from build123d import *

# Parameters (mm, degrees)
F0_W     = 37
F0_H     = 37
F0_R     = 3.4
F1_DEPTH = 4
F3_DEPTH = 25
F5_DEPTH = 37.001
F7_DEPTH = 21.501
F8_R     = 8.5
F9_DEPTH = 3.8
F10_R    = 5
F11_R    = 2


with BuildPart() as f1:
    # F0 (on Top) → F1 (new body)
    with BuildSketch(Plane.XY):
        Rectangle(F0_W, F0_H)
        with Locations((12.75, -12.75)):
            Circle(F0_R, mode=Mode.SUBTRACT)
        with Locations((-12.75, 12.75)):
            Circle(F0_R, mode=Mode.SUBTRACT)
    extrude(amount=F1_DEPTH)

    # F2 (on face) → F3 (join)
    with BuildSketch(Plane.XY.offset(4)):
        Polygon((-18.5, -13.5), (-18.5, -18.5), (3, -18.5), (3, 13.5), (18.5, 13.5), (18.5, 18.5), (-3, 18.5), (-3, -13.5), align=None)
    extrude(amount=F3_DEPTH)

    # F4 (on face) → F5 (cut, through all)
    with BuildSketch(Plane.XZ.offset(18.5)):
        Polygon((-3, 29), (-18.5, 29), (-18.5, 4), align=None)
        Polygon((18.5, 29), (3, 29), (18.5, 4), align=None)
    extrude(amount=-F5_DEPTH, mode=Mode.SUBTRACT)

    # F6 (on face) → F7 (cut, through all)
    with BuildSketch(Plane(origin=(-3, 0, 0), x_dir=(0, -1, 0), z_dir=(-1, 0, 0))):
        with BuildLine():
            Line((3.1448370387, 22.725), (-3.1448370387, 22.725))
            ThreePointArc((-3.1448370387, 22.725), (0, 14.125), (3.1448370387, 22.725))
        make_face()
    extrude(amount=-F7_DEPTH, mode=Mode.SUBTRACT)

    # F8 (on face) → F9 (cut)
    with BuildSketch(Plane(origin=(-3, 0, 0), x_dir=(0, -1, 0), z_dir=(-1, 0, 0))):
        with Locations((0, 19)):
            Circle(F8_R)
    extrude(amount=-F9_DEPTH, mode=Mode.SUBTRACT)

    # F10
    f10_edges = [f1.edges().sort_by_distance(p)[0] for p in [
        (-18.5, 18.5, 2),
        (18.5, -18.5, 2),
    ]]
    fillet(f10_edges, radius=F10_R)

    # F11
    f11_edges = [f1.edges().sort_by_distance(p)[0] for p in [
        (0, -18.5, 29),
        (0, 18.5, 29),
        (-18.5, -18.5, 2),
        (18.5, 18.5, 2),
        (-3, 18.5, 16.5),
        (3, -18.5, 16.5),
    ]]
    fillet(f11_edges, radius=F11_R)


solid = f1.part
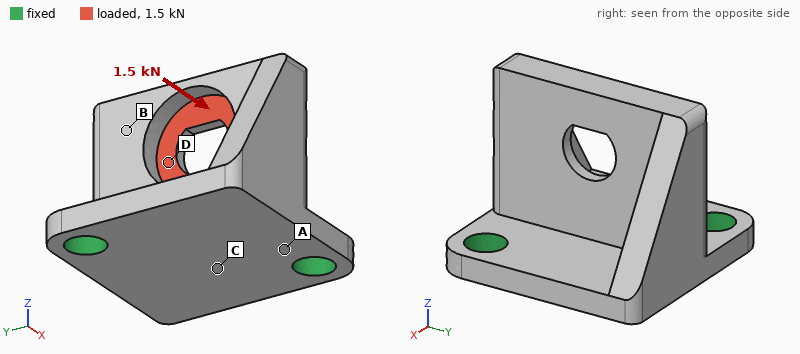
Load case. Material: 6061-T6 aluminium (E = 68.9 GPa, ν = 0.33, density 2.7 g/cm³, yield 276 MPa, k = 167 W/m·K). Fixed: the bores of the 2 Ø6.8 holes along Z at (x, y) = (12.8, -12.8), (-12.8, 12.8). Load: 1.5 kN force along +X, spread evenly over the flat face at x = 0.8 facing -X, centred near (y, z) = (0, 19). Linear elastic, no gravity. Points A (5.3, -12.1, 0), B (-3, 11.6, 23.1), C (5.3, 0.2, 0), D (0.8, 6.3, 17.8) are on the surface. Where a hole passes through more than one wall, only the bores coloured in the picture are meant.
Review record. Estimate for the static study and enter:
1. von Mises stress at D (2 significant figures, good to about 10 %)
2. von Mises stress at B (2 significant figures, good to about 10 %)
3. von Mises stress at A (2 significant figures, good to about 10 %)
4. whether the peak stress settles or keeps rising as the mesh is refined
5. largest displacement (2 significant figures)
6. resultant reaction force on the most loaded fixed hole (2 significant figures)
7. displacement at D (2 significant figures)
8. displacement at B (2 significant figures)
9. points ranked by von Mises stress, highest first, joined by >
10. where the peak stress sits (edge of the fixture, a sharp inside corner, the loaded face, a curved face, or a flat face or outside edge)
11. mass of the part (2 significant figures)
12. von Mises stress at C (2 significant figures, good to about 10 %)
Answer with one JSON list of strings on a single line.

["41 MPa", "21 MPa", "110 MPa", "keeps rising", "0.27 mm", "1.0 kN", "0.15 mm", "0.19 mm", "A > C > D > B", "edge of the fixture", "31 g", "70 MPa"]
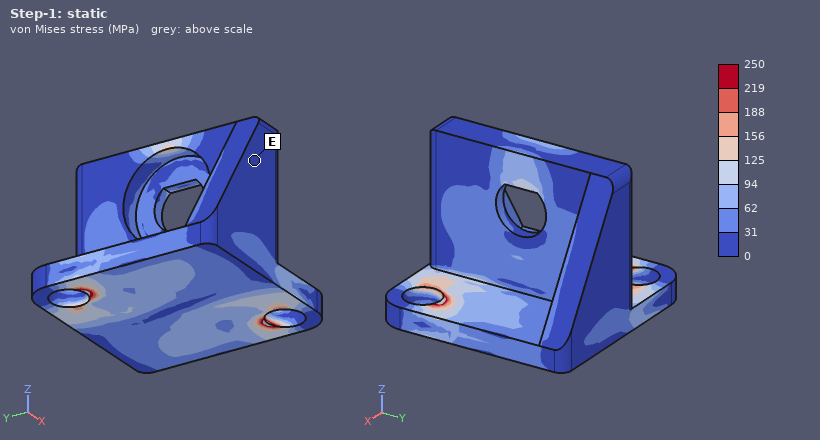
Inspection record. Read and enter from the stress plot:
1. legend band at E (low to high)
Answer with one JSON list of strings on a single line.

["0 to 31 MPa"]
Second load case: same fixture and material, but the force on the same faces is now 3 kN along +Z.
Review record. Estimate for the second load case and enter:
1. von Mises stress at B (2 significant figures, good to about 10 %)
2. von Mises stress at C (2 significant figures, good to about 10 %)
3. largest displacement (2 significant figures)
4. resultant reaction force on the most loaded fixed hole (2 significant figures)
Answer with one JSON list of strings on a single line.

["24 MPa", "46 MPa", "65 µm", "1.6 kN"]
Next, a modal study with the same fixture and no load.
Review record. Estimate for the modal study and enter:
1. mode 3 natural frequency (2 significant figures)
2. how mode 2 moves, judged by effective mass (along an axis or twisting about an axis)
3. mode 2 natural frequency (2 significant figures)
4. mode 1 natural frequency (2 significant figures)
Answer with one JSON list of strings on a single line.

["8300 Hz", "along Z", "7000 Hz", "3200 Hz"]
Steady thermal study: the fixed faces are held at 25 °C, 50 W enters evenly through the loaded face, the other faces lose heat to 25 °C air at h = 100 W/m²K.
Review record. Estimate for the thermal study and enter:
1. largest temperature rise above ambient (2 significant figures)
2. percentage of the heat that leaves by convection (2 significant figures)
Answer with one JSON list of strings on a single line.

["49 K", "21 %"]
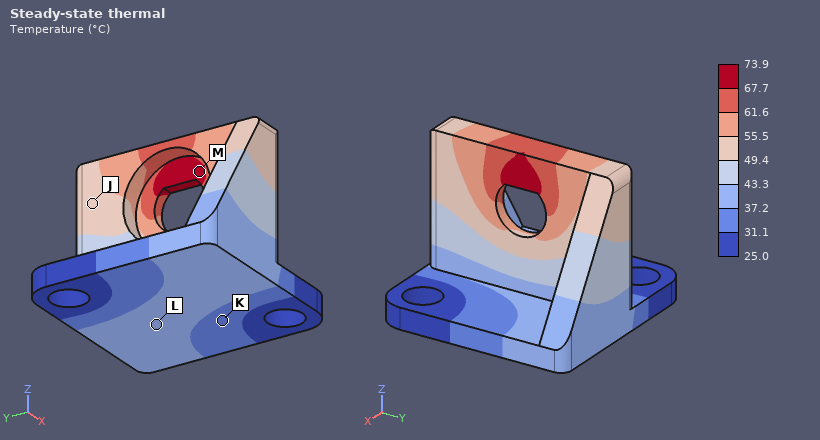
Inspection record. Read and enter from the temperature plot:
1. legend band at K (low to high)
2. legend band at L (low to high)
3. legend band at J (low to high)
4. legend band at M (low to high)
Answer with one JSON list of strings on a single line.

["31.1 to 37.2 °C", "37.2 to 43.3 °C", "49.4 to 55.5 °C", "67.7 to 73.9 °C"]
